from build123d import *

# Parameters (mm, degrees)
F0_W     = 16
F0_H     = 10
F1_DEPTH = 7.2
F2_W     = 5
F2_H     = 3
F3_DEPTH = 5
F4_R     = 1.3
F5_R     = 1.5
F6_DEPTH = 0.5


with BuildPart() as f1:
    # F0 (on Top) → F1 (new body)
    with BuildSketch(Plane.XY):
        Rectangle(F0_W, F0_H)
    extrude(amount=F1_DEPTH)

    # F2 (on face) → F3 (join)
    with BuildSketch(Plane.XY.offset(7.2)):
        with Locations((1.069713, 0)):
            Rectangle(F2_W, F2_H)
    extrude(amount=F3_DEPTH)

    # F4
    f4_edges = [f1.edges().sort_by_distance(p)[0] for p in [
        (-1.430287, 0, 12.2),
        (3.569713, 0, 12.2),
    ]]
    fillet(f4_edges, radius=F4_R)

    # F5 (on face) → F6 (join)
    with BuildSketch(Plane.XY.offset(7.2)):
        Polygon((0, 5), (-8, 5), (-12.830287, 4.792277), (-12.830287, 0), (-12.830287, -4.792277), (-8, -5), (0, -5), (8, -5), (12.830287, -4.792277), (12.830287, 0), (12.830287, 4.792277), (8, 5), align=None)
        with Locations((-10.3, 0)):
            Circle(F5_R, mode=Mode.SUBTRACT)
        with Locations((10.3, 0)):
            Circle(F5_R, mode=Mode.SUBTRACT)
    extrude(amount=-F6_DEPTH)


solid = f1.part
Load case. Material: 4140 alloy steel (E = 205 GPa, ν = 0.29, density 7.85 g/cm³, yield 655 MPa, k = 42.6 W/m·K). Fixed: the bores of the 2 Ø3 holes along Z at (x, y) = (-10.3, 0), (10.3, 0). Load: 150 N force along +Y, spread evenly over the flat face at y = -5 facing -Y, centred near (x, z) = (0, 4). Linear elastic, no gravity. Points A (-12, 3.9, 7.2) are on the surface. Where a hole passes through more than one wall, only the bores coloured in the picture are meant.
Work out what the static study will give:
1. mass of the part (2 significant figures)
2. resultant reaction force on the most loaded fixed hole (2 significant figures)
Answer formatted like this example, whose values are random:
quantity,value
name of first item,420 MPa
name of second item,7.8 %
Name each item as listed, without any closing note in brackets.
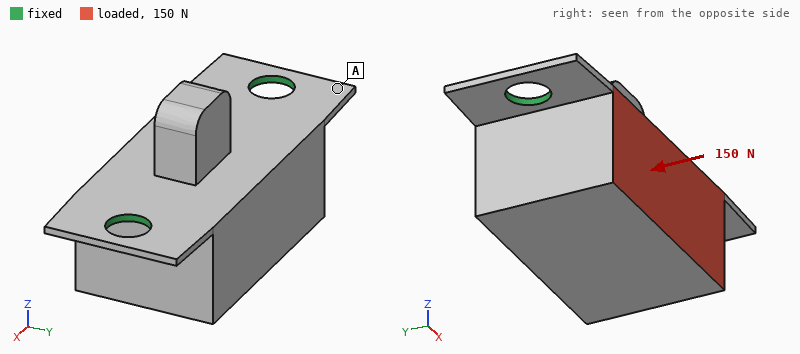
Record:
quantity,value
mass of the part,9.9 g
resultant reaction force on the most loaded fixed hole,75 N
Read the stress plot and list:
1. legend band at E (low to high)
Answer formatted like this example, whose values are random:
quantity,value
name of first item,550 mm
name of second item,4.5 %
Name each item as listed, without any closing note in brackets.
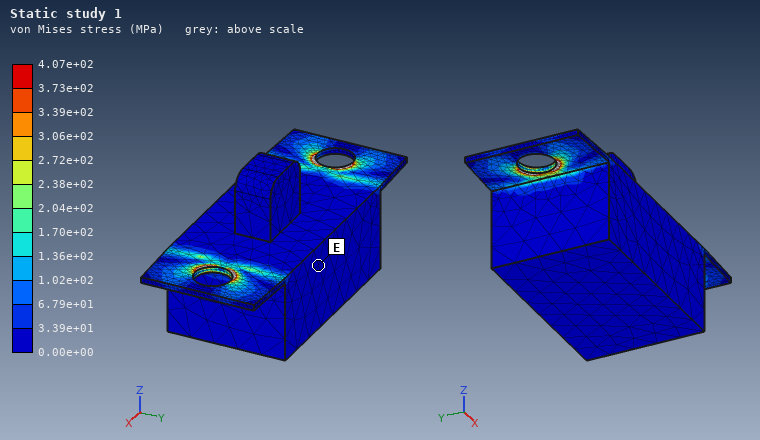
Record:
quantity,value
legend band at E,0.00e+00 to 3.39e+01 MPa
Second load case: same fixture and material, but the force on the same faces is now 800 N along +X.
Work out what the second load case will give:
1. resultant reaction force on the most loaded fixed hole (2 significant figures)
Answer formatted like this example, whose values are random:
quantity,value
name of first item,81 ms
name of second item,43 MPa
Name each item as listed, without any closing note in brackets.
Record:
quantity,value
resultant reaction force on the most loaded fixed hole,470 N
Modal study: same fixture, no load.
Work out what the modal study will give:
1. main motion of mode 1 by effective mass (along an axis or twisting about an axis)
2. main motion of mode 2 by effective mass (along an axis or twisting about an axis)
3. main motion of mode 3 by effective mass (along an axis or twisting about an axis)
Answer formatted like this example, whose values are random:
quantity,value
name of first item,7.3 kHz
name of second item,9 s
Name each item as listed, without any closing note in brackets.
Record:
quantity,value
main motion of mode 1 by effective mass,along Y
main motion of mode 2 by effective mass,along Z
main motion of mode 3 by effective mass,along X
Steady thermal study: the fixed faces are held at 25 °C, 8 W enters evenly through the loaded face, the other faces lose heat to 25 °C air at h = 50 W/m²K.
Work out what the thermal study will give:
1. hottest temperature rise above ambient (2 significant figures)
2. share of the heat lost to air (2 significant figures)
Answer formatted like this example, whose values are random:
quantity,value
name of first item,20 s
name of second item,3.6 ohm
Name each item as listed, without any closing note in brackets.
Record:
quantity,value
hottest temperature rise above ambient,52 K
share of the heat lost to air,19 %
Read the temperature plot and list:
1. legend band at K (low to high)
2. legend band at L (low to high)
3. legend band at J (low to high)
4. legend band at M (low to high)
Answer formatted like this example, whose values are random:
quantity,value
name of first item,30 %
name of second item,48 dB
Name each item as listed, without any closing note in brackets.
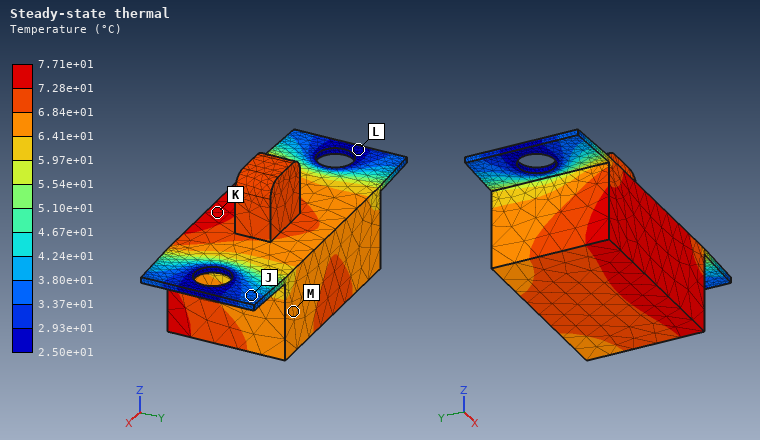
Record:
quantity,value
legend band at K,7.28e+01 to 7.71e+01 °C
legend band at L,2.50e+01 to 2.93e+01 °C
legend band at J,3.37e+01 to 3.80e+01 °C
legend band at M,6.41e+01 to 6.84e+01 °C
